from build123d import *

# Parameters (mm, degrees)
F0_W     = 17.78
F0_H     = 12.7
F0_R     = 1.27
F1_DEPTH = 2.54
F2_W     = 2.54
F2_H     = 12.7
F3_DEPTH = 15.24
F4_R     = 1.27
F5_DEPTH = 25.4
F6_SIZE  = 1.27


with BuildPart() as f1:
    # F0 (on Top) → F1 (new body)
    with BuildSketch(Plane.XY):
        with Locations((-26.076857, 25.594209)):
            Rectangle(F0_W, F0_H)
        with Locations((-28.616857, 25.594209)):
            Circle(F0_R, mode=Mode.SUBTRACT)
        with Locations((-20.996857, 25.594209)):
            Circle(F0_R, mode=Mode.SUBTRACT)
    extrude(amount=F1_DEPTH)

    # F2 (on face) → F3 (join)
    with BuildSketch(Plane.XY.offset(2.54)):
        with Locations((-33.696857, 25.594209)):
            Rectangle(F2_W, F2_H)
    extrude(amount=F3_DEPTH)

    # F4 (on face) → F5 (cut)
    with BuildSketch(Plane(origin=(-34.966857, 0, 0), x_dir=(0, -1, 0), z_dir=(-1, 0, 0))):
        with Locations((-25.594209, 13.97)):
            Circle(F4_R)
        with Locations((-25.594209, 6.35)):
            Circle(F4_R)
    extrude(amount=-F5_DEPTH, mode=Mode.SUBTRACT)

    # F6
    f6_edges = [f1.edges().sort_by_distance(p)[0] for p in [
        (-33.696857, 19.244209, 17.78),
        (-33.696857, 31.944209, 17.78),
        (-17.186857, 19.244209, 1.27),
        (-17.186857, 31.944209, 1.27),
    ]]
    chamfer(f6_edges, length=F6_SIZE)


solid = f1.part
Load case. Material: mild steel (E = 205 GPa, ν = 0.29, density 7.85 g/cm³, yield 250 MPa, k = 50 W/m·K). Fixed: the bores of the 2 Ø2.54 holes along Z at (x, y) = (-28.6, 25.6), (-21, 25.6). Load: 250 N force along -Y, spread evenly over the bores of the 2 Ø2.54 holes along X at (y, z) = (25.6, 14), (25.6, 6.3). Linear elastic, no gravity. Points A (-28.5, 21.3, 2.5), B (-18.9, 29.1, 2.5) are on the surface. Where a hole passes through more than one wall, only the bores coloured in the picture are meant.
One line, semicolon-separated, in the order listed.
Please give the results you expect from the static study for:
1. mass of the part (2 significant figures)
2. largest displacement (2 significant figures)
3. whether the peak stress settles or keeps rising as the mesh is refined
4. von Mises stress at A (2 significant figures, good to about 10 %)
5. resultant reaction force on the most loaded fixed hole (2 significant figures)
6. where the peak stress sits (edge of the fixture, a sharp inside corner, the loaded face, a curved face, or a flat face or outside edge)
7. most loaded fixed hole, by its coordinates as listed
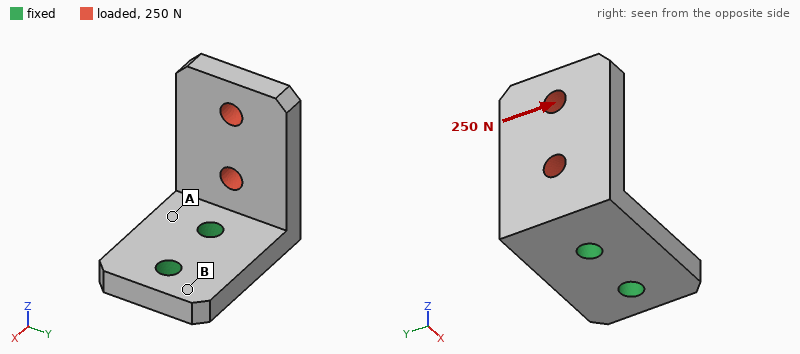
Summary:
7.9 g; 33 µm; keeps rising; 62 MPa; 350 N; edge of the fixture; (-28.6, 25.6)
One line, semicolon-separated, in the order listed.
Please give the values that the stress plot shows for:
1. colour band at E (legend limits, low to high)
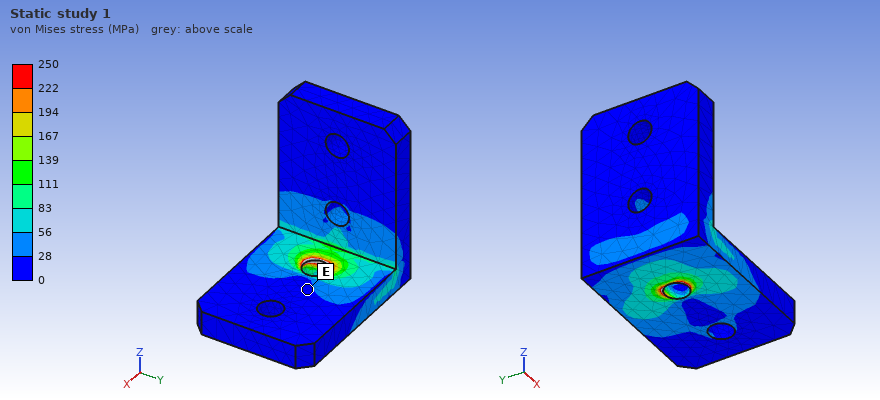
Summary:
0 to 28 MPa
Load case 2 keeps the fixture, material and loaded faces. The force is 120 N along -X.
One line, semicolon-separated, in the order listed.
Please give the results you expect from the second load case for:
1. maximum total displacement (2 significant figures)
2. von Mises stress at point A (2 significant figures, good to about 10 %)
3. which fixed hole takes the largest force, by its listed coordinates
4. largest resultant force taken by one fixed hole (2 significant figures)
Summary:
43 µm; 39 MPa; (-28.6, 25.6); 110 N
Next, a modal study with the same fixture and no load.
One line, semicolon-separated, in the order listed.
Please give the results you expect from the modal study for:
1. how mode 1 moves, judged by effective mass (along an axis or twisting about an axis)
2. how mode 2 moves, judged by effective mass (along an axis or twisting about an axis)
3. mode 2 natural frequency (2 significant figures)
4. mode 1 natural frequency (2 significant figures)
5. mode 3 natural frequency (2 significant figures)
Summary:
along X; along Y; 8500 Hz; 5400 Hz; 19 kHz
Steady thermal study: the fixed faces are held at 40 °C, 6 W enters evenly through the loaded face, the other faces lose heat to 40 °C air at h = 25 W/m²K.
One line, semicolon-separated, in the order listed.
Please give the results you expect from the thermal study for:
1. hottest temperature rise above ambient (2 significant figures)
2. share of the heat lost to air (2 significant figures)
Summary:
52 K; 9.0 %
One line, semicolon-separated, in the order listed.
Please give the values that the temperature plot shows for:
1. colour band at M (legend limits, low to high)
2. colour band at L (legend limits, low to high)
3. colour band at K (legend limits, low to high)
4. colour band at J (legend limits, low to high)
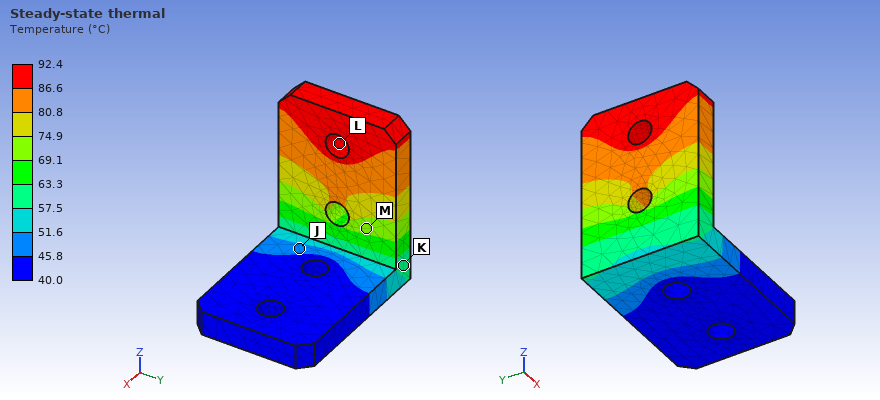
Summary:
69.1 to 74.9 °C; 86.6 to 92.4 °C; 57.5 to 63.3 °C; 45.8 to 51.6 °C
